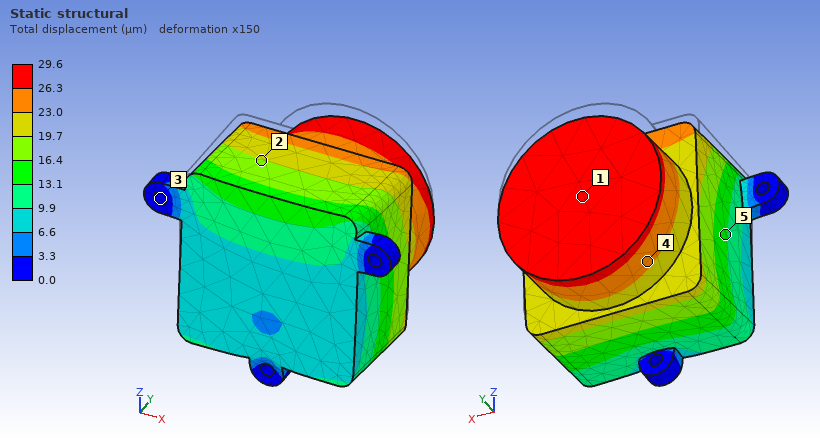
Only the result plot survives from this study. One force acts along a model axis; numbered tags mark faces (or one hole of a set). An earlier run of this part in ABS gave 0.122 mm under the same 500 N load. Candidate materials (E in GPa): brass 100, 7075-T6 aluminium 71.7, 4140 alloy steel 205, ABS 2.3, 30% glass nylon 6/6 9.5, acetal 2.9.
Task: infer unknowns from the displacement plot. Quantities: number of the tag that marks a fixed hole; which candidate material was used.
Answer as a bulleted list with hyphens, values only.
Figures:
- 3
- 30% glass nylon 6/6
